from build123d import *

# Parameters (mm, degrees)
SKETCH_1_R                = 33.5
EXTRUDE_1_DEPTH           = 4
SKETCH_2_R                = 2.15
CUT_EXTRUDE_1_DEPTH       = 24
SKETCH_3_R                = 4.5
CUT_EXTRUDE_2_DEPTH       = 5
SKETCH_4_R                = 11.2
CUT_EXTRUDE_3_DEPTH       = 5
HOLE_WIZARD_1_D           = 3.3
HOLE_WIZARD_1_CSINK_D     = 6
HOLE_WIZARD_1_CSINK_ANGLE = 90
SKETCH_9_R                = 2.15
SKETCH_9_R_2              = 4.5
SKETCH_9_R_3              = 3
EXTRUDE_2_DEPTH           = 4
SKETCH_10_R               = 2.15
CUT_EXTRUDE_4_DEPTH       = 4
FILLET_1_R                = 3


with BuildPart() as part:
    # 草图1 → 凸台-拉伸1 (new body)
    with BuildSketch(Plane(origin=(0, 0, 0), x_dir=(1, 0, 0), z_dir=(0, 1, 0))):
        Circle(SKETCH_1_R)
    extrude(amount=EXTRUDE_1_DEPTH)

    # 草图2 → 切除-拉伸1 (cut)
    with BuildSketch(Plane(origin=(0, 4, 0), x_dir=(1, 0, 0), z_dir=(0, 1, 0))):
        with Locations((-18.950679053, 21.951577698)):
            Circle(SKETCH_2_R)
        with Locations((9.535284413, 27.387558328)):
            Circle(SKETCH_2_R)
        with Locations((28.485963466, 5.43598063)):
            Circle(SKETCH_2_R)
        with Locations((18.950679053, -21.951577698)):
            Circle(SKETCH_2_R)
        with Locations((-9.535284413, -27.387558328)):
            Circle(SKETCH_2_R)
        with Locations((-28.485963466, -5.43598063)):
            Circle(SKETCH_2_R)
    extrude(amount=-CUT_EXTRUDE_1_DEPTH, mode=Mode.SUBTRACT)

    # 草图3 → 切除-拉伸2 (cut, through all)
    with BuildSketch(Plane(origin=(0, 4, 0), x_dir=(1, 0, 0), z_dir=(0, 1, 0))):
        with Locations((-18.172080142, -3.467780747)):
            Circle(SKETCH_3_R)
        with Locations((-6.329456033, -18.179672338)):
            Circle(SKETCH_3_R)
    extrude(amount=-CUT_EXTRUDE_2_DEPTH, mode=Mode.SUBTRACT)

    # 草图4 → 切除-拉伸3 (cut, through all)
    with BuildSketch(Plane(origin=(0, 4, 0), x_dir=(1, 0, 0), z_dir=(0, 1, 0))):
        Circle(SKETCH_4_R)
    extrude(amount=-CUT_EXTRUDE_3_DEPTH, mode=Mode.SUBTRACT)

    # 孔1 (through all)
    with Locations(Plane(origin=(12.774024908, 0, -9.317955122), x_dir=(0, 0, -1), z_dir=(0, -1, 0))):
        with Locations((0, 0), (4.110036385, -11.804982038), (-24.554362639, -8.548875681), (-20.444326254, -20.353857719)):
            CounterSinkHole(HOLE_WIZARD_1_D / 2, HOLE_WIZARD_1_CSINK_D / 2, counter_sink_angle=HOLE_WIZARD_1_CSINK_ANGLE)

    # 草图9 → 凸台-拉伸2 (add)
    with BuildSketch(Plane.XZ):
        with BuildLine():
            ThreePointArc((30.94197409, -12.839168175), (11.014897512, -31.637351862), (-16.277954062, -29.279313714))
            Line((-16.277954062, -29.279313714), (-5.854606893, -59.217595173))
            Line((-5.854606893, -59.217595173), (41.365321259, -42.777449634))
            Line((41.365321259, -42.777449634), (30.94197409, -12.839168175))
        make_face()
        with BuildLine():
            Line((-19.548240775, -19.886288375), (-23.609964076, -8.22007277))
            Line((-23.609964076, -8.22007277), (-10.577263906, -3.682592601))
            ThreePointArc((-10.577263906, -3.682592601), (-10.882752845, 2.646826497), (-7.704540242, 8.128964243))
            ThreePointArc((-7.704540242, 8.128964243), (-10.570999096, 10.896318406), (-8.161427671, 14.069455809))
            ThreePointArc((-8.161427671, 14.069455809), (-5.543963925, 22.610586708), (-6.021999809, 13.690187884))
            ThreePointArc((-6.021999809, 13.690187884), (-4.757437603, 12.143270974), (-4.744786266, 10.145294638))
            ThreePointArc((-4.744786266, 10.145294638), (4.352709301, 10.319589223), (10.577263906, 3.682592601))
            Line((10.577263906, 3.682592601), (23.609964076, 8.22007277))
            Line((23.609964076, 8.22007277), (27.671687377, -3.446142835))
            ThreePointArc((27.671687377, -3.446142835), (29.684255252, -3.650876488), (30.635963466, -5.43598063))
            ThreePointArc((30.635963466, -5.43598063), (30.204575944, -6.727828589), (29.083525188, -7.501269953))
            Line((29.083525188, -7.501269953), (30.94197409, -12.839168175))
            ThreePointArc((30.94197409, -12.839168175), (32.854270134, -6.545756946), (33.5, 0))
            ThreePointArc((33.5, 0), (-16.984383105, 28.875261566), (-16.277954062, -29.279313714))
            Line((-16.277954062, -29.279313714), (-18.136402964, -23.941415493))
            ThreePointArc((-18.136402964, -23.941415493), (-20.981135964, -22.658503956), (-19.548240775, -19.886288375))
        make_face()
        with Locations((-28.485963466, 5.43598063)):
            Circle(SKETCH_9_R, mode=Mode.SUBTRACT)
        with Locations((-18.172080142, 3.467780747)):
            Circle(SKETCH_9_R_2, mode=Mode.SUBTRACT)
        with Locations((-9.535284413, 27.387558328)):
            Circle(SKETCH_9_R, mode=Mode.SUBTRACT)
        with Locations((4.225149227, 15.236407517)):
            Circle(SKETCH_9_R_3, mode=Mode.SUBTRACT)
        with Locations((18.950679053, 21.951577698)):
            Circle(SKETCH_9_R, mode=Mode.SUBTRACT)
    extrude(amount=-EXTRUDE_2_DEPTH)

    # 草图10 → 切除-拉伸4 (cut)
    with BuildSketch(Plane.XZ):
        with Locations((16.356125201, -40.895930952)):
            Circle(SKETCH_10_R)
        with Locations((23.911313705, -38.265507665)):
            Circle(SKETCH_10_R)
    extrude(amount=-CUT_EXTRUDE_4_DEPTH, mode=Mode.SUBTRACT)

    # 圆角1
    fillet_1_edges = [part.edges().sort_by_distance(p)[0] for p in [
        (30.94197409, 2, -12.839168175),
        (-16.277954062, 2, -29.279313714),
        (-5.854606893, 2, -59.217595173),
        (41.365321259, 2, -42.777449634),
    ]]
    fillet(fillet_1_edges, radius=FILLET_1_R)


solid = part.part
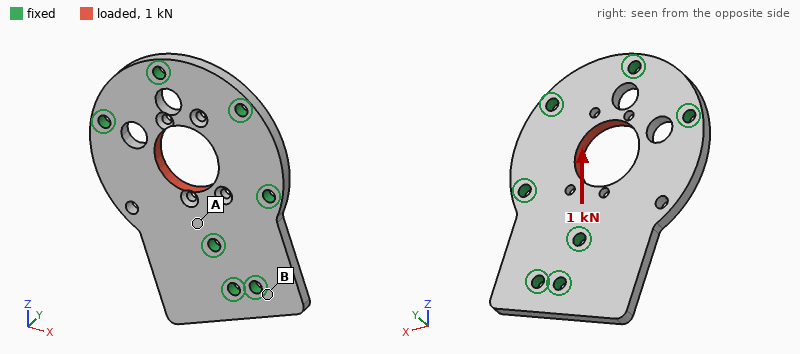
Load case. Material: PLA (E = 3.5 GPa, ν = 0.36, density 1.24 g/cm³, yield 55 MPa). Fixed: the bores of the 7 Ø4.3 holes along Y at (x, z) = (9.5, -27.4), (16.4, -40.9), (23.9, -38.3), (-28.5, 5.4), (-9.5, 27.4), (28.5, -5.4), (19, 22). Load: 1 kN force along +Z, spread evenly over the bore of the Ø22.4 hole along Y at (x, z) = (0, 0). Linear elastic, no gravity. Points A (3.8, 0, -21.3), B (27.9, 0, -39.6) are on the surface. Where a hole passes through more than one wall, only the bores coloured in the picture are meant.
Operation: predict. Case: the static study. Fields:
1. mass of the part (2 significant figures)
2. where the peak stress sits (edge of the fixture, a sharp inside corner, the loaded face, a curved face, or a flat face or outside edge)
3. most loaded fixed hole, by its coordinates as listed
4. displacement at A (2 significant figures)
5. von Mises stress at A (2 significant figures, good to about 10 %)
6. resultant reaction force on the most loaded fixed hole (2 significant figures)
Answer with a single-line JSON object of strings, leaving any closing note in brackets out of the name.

{"mass of the part": "20 g", "where the peak stress sits": "the loaded face", "most loaded fixed hole, by its coordinates as listed": "(9.5, -27.4)", "displacement at A": "16 µm", "von Mises stress at A": "4.0 MPa", "resultant reaction force on the most loaded fixed hole": "270 N"}
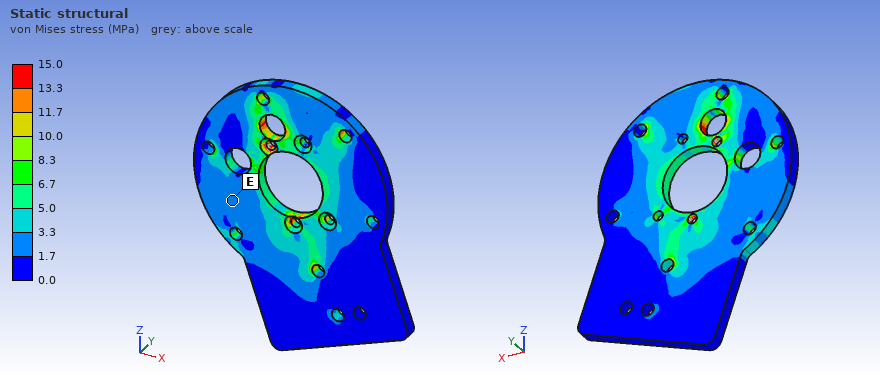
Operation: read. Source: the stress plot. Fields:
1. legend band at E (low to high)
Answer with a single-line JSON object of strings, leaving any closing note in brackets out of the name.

{"legend band at E": "1.7 to 3.3 MPa"}
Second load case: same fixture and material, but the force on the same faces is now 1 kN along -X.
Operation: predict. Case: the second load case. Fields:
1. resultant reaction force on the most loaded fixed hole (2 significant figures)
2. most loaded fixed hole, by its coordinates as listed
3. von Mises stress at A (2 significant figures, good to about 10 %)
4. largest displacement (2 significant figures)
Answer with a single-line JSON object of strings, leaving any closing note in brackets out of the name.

{"resultant reaction force on the most loaded fixed hole": "290 N", "most loaded fixed hole, by its coordinates as listed": "(28.5, -5.4)", "von Mises stress at A": "3.5 MPa", "largest displacement": "61 µm"}
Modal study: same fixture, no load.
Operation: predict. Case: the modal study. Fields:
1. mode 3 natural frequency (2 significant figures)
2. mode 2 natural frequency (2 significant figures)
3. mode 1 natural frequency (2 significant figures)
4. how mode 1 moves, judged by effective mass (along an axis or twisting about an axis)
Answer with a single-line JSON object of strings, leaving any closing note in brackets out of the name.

{"mode 3 natural frequency": "3800 Hz", "mode 2 natural frequency": "2500 Hz", "mode 1 natural frequency": "1700 Hz", "how mode 1 moves, judged by effective mass": "along Y"}
